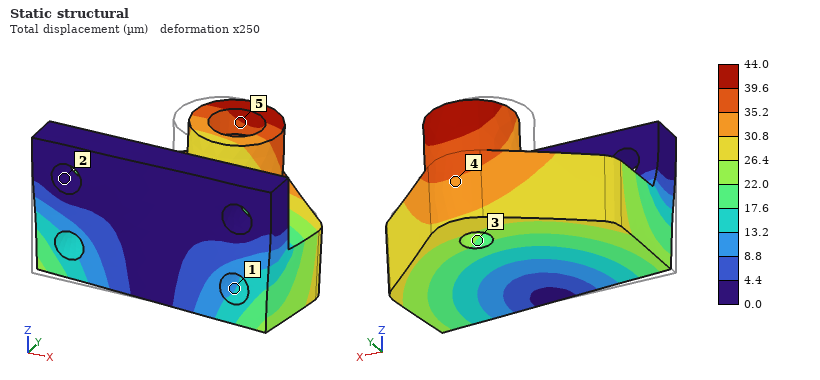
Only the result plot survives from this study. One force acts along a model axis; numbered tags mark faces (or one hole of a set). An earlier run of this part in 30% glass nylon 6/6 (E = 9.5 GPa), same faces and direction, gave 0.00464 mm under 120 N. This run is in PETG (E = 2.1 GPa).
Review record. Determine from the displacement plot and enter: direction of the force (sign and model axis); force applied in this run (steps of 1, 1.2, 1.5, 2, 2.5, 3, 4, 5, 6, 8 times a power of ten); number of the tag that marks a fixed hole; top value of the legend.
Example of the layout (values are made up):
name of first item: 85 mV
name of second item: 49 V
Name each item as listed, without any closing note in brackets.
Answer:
direction of the force: +X
force applied in this run: 250 N
number of the tag that marks a fixed hole: 2
top value of the legend: 44.0 µm
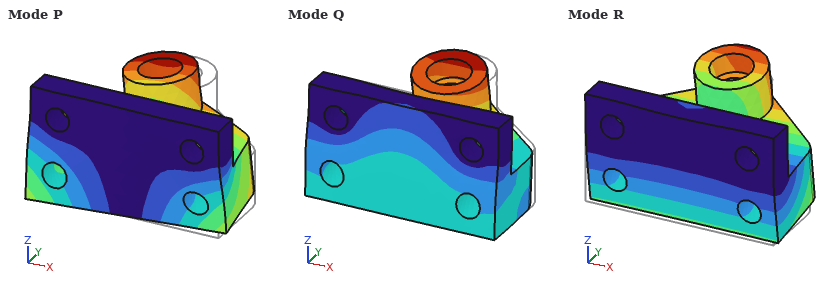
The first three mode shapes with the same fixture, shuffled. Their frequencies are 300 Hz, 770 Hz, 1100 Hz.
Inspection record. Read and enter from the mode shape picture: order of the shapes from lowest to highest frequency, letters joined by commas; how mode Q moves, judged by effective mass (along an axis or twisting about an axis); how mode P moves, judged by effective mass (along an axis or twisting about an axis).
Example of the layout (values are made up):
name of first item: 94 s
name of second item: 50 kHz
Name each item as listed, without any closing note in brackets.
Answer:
order of the shapes from lowest to highest frequency, letters joined by commas: R, P, Q
how mode Q moves, judged by effective mass: along Y
how mode P moves, judged by effective mass: along X
